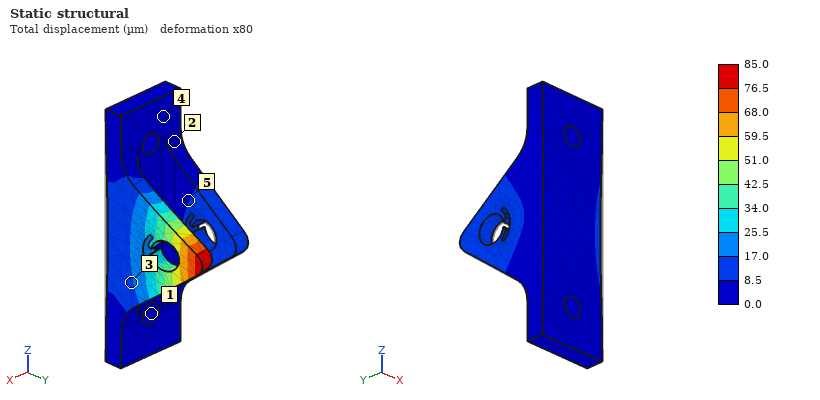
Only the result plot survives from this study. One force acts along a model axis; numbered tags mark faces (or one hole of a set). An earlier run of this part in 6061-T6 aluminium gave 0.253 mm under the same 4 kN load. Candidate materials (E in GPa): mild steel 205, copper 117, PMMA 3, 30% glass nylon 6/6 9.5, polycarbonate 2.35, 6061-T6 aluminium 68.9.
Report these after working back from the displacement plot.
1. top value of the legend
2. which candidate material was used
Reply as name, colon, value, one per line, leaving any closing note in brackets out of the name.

top value of the legend: 85.0 µm
which candidate material was used: mild steel
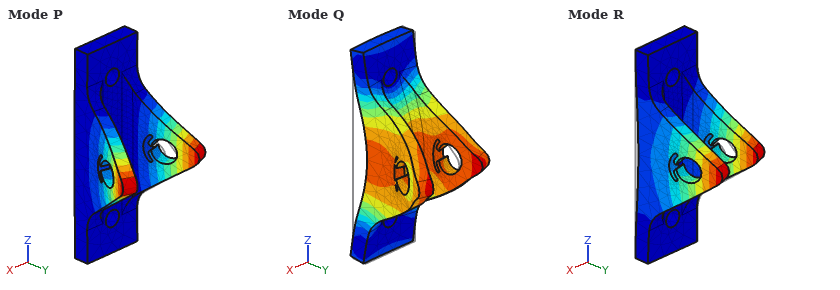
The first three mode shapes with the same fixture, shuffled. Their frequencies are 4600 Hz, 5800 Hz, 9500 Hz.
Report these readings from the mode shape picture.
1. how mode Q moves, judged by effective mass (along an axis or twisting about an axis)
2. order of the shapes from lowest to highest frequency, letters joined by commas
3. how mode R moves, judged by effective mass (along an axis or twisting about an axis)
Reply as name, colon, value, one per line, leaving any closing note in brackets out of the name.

how mode Q moves, judged by effective mass: along Y
order of the shapes from lowest to highest frequency, letters joined by commas: R, P, Q
how mode R moves, judged by effective mass: along X
